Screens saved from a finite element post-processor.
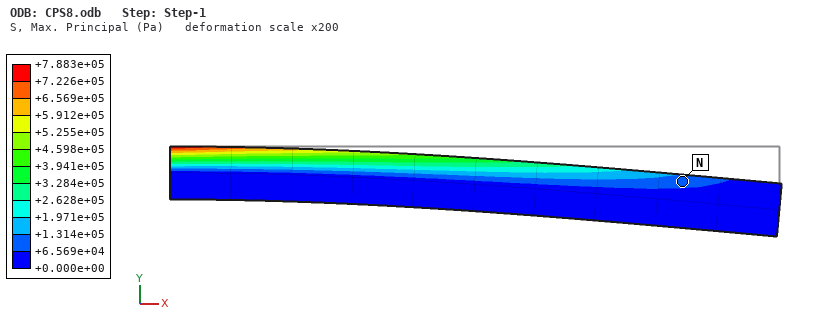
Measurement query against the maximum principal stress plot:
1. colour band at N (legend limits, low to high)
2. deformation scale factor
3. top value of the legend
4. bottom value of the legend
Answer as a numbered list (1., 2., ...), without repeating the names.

1. +6.569e+04 to +1.314e+05 Pa
2. 200
3. +7.883e+05 Pa
4. +0.000e+00 Pa
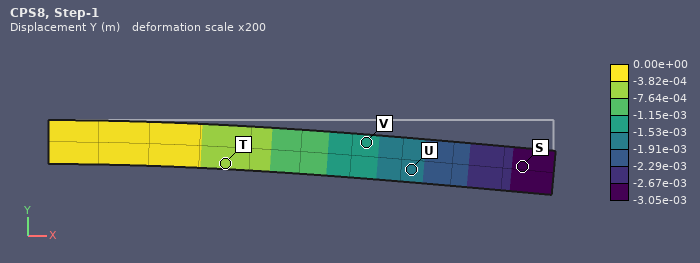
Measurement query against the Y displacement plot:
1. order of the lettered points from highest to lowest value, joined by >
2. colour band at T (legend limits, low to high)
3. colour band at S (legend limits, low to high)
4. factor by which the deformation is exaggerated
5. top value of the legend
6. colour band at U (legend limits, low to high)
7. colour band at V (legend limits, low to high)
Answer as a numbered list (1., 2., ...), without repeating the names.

1. T > V > U > S
2. -7.64e-04 to -3.82e-04 m
3. -3.05e-03 to -2.67e-03 m
4. 200
5. 0.00e+00 m
6. -1.91e-03 to -1.53e-03 m
7. -1.53e-03 to -1.15e-03 m
